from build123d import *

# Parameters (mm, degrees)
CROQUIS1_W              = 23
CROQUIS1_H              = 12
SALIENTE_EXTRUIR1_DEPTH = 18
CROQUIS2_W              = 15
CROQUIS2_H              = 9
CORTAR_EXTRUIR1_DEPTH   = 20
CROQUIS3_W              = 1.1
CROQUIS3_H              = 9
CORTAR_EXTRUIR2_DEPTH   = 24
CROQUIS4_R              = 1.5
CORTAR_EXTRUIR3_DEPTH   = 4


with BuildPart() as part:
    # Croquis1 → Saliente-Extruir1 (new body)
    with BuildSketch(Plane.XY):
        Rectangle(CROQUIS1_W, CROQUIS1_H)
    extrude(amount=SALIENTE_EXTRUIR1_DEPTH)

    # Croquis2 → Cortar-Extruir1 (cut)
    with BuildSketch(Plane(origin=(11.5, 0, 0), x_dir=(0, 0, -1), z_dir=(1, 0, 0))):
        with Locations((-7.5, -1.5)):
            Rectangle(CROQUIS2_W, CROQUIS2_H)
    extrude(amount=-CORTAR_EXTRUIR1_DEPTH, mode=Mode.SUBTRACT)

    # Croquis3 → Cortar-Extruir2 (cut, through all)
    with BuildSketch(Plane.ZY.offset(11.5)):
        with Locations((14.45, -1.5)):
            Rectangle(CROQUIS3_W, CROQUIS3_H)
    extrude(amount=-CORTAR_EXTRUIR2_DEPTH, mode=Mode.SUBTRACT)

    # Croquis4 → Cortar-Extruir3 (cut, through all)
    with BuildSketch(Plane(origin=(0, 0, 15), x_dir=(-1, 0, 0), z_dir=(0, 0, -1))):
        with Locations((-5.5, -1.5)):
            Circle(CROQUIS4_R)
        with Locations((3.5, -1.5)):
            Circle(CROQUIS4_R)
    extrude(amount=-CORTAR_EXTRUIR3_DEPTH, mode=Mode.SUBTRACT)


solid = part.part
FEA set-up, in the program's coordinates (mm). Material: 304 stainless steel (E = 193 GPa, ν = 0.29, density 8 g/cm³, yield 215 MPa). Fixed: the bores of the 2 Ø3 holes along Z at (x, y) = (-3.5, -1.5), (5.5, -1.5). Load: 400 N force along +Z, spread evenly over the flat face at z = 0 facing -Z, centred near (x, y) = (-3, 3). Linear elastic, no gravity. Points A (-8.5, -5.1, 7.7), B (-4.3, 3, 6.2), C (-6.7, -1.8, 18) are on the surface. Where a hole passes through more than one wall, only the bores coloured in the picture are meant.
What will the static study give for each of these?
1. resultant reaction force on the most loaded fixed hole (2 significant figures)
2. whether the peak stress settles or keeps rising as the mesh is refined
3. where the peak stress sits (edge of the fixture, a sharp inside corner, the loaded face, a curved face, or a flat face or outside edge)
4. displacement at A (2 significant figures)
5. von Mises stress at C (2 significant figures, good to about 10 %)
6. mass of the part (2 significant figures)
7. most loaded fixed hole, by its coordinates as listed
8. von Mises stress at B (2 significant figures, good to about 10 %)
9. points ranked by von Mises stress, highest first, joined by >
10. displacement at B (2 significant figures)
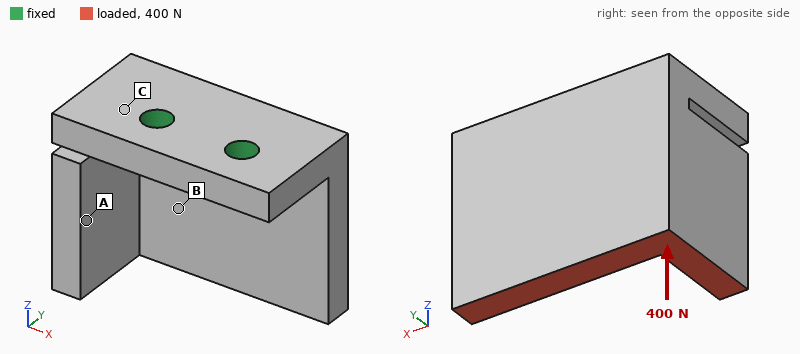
310 N
keeps rising
edge of the fixture
5.7 µm
24 MPa
18 g
(-3.5, -1.5)
13 MPa
C > B > A
3.5 µm
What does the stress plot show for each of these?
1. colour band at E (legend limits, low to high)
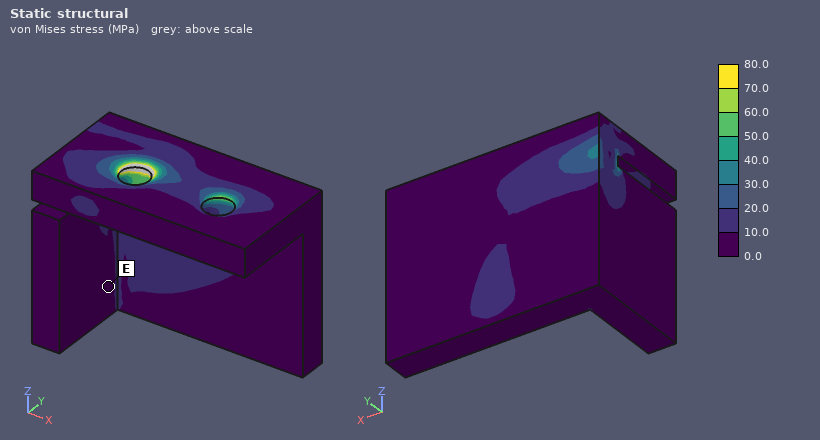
0.0 to 10.0 MPa
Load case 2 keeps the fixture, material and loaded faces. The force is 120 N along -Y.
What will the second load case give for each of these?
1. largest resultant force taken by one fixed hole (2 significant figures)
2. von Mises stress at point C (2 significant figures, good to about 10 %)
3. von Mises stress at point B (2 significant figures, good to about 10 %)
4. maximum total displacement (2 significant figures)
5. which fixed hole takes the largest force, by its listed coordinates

100 N
25 MPa
9.6 MPa
38 µm
(-3.5, -1.5)
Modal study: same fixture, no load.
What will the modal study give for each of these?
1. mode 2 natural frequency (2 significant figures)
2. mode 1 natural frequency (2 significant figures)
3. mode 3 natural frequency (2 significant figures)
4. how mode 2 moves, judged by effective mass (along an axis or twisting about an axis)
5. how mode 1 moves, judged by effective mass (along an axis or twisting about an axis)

8200 Hz
4700 Hz
11 kHz
along X
along Y
